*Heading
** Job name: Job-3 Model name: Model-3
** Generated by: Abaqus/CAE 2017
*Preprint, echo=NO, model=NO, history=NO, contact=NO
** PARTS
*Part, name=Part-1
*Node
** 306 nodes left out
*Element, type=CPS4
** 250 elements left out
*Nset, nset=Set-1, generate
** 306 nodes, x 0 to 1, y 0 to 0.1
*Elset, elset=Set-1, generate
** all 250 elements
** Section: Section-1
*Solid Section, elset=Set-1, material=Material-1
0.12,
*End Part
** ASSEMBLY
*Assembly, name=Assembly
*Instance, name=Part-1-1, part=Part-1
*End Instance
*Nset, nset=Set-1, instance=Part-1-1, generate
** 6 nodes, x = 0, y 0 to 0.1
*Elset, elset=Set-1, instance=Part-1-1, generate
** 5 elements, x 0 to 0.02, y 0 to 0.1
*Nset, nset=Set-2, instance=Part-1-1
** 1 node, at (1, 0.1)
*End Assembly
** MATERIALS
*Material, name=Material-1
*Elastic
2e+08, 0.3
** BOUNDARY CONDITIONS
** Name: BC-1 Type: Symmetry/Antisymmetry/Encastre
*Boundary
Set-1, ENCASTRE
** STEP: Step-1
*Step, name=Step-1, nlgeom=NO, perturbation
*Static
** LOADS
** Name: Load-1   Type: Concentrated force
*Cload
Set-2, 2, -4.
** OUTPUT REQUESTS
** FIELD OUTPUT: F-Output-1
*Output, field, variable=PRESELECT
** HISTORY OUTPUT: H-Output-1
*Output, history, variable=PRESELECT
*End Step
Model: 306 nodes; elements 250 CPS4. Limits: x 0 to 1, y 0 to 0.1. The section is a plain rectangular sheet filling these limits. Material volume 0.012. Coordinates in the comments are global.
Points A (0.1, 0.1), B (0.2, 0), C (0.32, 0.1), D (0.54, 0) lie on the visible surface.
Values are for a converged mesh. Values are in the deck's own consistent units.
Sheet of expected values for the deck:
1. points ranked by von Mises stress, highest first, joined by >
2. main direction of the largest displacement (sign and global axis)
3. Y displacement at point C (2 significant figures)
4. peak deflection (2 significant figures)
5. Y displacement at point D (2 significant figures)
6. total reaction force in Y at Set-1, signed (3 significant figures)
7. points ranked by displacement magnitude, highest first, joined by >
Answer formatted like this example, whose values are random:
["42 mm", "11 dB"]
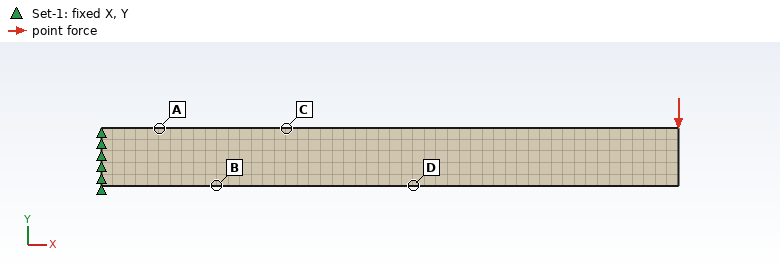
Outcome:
["A > B > C > D", "-Y", "-9.0e-05", "6.5e-04", "-2.3e-04", "4.00", "D > C > B > A"]
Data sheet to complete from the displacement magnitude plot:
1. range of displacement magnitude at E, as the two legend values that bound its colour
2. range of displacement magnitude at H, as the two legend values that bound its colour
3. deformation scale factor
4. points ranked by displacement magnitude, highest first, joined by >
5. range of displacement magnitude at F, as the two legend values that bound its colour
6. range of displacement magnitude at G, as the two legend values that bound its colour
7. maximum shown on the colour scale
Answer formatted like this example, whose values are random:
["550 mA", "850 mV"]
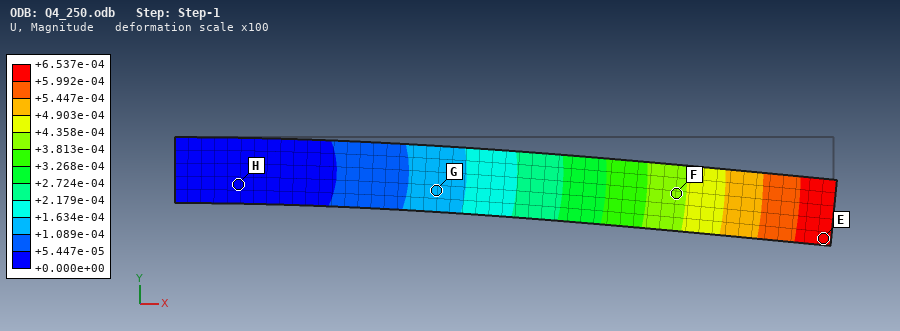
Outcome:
["+5.992e-04 to +6.537e-04", "+0.000e+00 to +5.447e-05", "100", "E > F > G > H", "+3.813e-04 to +4.358e-04", "+1.089e-04 to +1.634e-04", "+6.537e-04"]
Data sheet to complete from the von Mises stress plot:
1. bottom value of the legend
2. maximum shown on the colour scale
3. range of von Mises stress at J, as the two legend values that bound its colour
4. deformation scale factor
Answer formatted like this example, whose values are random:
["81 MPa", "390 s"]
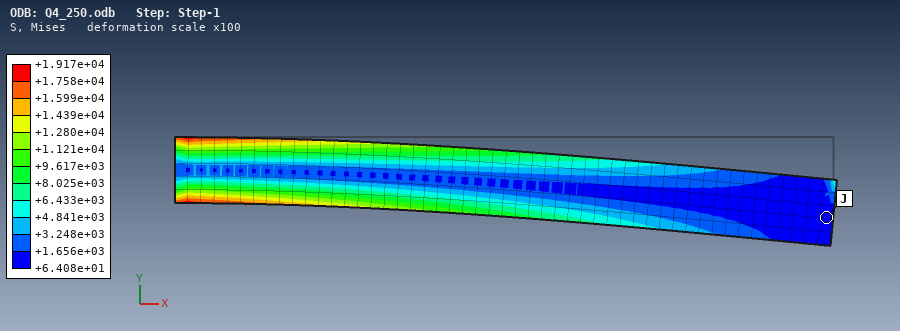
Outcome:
["+6.408e+01", "+1.917e+04", "+6.408e+01 to +1.656e+03", "100"]
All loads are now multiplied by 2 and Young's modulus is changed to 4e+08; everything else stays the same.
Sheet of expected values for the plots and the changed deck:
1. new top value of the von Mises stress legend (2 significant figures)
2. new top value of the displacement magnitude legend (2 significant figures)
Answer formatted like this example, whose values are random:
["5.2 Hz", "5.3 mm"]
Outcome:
["38000", "6.5e-04"]
